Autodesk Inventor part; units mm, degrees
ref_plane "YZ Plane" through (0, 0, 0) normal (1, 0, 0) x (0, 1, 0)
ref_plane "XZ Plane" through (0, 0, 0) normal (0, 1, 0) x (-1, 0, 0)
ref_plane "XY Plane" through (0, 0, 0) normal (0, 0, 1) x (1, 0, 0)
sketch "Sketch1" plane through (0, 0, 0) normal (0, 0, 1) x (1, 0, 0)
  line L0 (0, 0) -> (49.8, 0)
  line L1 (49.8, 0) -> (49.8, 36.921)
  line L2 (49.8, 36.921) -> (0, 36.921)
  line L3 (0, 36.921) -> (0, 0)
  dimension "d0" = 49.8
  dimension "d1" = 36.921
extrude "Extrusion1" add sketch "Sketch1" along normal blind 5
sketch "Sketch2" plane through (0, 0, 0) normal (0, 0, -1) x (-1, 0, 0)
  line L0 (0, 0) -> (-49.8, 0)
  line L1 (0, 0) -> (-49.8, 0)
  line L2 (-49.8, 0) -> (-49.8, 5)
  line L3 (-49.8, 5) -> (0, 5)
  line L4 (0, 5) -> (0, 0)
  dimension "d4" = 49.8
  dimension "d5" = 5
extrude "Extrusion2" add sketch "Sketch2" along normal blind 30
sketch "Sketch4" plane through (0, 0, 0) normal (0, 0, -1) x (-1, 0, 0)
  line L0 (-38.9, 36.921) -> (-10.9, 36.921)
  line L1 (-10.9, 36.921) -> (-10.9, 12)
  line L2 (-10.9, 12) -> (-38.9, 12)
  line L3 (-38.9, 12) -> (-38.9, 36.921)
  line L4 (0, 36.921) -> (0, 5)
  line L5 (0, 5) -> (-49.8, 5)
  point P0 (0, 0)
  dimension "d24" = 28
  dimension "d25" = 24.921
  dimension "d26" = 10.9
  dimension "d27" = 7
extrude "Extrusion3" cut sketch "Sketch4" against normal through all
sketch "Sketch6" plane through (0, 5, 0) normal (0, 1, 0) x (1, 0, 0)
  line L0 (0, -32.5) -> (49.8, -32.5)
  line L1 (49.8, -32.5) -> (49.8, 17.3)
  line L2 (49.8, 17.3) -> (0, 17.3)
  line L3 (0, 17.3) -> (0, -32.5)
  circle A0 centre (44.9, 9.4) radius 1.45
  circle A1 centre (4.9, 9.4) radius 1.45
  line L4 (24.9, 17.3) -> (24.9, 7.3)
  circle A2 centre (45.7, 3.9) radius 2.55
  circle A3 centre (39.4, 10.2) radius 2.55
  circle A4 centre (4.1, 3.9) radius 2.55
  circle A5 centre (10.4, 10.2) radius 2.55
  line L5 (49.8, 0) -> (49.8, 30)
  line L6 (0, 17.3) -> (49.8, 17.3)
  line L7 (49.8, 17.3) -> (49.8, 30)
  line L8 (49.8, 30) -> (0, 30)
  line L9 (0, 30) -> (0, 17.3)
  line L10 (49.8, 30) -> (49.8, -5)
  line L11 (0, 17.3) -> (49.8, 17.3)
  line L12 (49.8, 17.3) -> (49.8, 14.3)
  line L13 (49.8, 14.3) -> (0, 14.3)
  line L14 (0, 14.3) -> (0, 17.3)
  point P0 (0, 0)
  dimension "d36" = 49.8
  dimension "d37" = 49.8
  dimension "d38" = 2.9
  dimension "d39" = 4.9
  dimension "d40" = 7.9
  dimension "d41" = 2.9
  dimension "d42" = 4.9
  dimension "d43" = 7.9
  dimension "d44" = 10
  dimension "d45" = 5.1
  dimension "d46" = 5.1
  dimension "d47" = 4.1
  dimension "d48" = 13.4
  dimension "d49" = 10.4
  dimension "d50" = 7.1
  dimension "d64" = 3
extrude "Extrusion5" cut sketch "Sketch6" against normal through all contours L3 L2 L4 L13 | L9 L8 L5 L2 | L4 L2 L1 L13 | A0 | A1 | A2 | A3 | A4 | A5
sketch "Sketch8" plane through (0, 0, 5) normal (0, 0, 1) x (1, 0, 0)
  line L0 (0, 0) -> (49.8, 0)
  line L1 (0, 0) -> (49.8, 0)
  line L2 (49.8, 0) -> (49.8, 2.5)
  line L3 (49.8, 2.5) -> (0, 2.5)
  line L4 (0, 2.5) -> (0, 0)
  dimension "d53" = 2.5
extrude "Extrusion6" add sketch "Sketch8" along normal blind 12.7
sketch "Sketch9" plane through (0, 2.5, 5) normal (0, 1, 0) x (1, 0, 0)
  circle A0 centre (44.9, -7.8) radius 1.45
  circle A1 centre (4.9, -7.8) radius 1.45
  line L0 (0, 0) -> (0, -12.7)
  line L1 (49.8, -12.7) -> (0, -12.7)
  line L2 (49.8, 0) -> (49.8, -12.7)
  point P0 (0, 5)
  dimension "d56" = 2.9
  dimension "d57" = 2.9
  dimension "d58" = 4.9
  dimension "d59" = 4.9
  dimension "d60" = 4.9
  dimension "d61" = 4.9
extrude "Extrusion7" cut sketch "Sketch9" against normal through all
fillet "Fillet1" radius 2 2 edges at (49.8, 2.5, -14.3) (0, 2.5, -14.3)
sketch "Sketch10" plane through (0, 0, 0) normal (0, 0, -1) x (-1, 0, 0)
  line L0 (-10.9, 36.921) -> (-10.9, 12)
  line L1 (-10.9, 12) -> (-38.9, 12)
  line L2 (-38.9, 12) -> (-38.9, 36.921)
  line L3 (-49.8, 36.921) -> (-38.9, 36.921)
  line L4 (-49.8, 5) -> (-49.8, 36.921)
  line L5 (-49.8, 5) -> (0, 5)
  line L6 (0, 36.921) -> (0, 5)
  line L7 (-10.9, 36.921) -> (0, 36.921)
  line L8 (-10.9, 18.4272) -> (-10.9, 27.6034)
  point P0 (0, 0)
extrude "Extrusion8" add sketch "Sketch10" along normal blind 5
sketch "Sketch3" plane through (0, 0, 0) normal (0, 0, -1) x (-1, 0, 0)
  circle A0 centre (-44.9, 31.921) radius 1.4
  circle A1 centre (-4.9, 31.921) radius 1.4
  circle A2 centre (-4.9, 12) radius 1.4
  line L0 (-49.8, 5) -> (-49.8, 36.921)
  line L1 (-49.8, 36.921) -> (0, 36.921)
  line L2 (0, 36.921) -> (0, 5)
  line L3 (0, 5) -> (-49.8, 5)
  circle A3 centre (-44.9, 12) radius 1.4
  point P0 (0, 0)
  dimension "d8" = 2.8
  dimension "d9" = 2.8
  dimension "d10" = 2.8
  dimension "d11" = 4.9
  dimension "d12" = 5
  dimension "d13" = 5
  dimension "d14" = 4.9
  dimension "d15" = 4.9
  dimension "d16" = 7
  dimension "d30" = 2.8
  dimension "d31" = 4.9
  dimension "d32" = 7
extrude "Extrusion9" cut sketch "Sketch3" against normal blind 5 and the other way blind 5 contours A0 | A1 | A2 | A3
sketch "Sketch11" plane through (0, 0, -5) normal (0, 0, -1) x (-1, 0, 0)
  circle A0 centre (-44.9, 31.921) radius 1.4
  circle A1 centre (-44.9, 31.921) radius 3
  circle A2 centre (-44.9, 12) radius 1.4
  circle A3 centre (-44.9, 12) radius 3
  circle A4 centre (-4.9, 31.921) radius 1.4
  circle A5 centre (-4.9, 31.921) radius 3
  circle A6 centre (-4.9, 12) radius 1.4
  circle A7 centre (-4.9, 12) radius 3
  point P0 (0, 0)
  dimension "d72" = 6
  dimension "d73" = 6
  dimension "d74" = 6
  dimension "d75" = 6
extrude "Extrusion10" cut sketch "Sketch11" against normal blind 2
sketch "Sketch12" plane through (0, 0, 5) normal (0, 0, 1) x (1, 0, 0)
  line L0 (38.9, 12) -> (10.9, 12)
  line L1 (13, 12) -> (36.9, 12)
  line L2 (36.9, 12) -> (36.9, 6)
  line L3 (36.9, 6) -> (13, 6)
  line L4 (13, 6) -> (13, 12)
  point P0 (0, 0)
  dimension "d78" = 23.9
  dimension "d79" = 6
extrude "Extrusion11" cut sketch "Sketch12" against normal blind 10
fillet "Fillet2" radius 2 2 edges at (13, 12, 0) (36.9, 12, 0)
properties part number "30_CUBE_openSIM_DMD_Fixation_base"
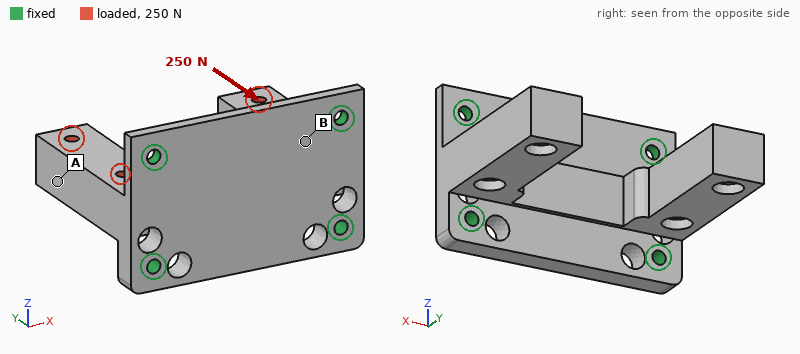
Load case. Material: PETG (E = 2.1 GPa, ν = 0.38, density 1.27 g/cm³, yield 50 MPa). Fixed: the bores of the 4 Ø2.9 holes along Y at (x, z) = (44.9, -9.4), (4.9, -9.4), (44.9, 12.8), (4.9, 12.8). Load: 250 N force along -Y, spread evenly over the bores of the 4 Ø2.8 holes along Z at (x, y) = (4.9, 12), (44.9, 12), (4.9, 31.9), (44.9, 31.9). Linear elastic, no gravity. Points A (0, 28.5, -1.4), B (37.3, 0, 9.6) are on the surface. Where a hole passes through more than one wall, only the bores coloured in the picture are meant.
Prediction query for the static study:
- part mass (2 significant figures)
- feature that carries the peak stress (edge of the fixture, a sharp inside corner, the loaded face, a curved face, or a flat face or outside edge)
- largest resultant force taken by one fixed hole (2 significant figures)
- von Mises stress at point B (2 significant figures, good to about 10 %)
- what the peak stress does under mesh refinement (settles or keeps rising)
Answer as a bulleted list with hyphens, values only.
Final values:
- 16 g
- edge of the fixture
- 73 N
- 2.8 MPa
- keeps rising
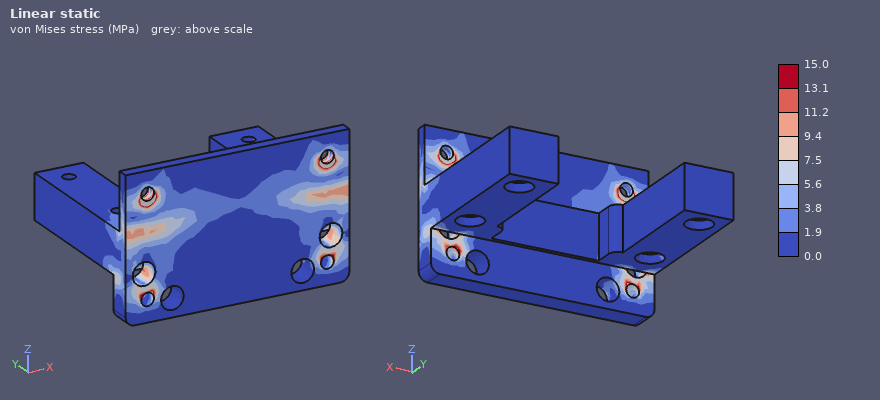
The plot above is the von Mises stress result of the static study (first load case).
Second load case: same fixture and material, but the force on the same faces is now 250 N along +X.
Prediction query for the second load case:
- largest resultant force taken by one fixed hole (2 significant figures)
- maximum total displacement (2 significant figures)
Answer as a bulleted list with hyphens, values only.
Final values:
- 120 N
- 0.72 mm
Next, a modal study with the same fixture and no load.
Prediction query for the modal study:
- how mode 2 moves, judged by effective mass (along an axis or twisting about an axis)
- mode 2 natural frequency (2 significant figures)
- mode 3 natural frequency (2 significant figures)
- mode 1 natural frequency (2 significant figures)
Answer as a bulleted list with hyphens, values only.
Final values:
- along Z
- 1100 Hz
- 1100 Hz
- 1000 Hz
